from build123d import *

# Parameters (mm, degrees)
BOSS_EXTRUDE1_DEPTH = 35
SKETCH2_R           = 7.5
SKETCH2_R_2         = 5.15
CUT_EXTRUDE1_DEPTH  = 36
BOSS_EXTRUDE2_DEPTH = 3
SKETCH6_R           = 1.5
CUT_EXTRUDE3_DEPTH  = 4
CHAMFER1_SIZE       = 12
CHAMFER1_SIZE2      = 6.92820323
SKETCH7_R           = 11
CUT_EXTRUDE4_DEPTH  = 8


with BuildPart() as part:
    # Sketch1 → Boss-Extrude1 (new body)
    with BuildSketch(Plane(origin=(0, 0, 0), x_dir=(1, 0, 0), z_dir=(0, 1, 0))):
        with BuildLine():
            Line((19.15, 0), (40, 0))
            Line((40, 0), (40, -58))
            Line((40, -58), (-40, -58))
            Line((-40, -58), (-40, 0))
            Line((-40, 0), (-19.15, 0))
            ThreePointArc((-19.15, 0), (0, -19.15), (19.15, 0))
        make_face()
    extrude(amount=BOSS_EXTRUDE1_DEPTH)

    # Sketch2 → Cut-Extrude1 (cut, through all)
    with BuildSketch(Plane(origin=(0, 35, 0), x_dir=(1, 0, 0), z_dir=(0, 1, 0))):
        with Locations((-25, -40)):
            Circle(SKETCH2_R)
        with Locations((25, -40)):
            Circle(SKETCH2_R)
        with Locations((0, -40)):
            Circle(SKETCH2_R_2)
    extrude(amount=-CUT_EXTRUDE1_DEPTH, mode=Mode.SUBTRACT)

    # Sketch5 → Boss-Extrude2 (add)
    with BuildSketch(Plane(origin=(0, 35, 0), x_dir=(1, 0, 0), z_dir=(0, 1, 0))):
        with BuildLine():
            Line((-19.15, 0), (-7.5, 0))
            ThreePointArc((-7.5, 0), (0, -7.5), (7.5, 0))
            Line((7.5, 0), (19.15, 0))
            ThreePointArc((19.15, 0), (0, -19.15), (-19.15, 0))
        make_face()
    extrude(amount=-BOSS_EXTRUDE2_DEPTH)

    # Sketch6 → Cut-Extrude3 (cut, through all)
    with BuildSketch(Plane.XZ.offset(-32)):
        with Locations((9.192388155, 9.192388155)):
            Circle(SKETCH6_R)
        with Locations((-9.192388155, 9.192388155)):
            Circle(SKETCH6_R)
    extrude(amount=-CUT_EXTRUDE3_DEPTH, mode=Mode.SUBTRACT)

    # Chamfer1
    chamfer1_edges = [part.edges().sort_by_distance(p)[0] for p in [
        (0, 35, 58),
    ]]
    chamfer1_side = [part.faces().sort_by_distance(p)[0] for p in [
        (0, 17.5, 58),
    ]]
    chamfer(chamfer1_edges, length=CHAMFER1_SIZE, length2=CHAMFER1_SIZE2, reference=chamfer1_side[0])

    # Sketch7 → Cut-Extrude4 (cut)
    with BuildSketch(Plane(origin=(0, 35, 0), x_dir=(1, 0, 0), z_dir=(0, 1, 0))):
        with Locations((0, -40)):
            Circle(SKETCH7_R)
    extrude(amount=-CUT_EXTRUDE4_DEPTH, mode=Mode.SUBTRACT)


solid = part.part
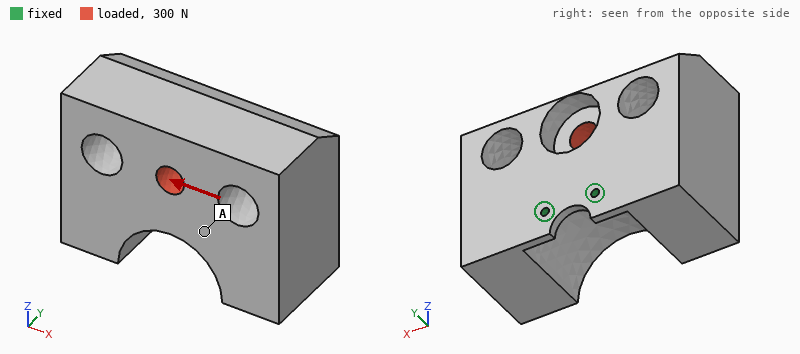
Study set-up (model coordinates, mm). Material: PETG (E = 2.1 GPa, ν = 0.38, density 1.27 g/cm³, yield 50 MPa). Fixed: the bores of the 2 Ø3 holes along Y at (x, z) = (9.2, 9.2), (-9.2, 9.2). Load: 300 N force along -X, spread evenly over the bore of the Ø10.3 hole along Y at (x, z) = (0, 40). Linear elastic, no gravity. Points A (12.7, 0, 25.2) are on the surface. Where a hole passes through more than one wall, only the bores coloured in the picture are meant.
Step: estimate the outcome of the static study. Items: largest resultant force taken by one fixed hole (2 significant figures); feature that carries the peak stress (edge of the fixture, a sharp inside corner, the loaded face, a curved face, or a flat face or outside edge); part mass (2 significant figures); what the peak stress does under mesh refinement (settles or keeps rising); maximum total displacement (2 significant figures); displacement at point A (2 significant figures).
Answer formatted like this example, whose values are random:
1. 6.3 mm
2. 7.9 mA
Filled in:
1. 540 N
2. edge of the fixture
3. 160 g
4. keeps rising
5. 1.00 mm
6. 0.62 mm
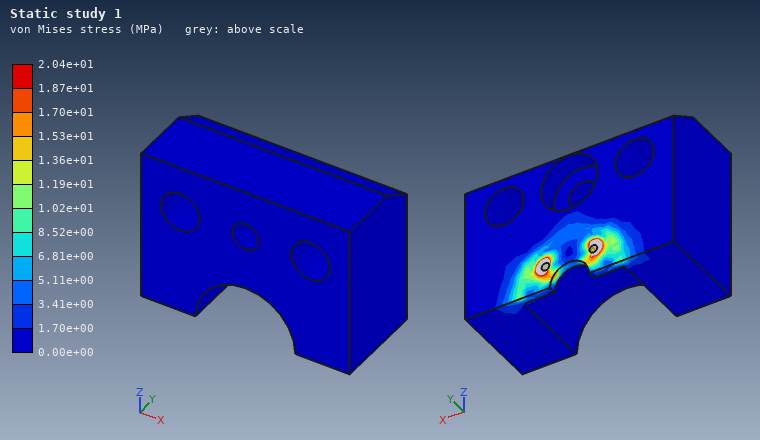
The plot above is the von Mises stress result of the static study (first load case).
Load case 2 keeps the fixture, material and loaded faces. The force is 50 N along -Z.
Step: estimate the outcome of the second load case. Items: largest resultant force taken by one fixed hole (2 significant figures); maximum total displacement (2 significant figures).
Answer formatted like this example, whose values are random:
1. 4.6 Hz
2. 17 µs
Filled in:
1. 27 N
2. 1.2 mm
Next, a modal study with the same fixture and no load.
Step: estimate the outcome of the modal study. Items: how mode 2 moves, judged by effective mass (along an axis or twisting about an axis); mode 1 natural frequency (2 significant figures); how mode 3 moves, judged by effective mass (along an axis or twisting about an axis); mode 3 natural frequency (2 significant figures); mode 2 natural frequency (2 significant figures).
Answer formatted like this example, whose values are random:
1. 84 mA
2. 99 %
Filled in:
1. along X
2. 89 Hz
3. along X
4. 400 Hz
5. 250 Hz
